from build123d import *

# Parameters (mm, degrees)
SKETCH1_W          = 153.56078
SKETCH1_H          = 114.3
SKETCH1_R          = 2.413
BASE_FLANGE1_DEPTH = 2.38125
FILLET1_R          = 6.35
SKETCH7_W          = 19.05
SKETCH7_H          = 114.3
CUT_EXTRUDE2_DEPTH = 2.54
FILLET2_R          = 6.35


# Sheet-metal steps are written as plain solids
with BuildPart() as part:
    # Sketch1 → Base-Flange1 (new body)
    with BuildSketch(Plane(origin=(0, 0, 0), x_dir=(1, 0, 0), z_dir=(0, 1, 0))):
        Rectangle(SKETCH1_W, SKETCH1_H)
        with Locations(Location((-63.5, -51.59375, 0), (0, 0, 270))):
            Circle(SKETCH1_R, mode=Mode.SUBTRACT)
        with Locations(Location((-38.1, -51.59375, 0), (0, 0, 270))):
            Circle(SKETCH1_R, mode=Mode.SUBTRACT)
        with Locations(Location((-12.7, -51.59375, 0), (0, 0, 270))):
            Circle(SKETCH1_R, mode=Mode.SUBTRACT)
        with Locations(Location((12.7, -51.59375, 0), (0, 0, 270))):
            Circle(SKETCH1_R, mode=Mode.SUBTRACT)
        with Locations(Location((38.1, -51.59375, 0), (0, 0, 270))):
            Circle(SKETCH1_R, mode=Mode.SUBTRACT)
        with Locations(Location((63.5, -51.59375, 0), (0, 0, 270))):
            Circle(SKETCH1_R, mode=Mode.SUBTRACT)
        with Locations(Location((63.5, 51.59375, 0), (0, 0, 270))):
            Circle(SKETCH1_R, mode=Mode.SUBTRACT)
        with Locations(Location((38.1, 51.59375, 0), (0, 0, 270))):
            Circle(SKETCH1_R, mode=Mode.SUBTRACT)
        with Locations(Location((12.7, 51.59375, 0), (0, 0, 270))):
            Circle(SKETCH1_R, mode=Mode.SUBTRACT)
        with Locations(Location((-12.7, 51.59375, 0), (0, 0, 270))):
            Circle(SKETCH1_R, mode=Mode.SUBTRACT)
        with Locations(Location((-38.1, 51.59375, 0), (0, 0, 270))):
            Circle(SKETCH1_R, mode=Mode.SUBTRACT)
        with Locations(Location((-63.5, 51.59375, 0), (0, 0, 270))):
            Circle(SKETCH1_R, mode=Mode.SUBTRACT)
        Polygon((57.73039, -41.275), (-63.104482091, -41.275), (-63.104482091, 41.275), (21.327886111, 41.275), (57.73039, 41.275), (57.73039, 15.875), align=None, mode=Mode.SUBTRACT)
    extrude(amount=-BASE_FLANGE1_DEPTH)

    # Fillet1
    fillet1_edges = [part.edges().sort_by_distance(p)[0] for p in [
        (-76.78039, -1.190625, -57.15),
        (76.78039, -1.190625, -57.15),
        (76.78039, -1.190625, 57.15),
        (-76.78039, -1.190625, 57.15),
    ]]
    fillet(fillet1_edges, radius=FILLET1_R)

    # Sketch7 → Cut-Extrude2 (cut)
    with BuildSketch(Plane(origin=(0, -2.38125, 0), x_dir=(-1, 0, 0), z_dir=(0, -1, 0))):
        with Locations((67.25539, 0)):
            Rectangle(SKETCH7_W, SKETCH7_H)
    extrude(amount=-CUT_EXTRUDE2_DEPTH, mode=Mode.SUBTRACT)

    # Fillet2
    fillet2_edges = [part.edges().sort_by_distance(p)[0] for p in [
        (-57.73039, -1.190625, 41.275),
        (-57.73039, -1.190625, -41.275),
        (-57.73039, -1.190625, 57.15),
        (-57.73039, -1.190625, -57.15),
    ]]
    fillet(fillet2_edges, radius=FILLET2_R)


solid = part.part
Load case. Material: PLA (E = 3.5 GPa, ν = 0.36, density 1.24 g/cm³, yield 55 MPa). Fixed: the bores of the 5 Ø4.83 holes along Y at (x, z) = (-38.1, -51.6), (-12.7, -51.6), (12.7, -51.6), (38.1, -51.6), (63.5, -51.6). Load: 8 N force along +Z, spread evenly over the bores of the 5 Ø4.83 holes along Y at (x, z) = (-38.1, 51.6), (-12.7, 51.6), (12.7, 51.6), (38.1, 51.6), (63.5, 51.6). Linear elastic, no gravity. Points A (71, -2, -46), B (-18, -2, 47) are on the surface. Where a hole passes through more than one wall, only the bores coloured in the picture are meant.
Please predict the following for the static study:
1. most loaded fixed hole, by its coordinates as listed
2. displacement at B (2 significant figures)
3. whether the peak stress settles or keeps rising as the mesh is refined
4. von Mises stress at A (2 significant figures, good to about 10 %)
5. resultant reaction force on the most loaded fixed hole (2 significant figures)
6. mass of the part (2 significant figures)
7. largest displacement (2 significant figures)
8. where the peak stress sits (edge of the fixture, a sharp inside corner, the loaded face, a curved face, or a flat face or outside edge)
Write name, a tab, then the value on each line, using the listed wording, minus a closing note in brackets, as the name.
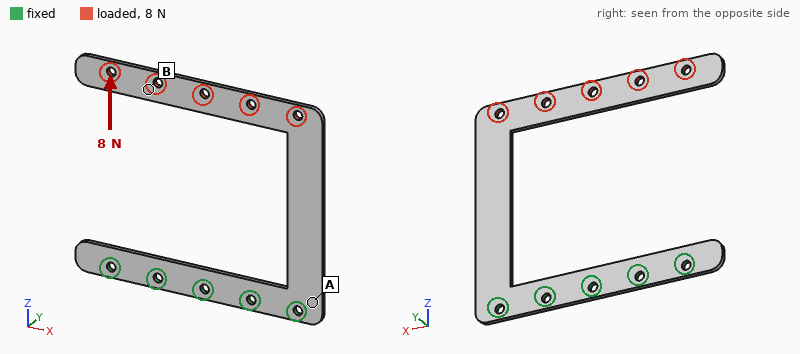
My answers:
most loaded fixed hole, by its coordinates as listed	(38.1, -51.6)
displacement at B	1.2 mm
whether the peak stress settles or keeps rising as the mesh is refined	keeps rising
von Mises stress at A	1.6 MPa
resultant reaction force on the most loaded fixed hole	16 N
mass of the part	17 g
largest displacement	1.8 mm
where the peak stress sits	a sharp inside corner
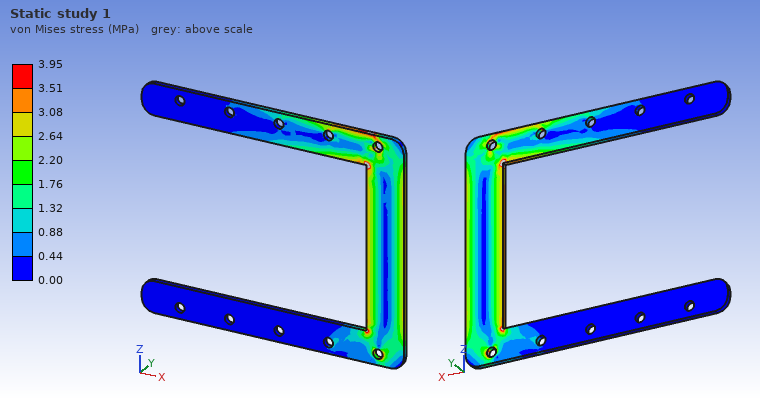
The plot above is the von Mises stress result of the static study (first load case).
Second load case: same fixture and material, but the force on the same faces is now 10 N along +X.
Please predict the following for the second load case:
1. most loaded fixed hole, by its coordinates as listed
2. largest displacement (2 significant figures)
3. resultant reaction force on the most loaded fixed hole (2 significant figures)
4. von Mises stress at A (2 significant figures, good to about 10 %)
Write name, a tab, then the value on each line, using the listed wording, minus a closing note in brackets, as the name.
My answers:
most loaded fixed hole, by its coordinates as listed	(38.1, -51.6)
largest displacement	1.8 mm
resultant reaction force on the most loaded fixed hole	39 N
von Mises stress at A	3.7 MPa
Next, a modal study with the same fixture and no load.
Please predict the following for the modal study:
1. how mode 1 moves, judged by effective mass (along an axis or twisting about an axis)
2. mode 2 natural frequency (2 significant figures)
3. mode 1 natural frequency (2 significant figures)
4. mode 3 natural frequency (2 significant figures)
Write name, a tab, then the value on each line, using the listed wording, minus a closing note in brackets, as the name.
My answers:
how mode 1 moves, judged by effective mass	along Y
mode 2 natural frequency	54 Hz
mode 1 natural frequency	21 Hz
mode 3 natural frequency	140 Hz
